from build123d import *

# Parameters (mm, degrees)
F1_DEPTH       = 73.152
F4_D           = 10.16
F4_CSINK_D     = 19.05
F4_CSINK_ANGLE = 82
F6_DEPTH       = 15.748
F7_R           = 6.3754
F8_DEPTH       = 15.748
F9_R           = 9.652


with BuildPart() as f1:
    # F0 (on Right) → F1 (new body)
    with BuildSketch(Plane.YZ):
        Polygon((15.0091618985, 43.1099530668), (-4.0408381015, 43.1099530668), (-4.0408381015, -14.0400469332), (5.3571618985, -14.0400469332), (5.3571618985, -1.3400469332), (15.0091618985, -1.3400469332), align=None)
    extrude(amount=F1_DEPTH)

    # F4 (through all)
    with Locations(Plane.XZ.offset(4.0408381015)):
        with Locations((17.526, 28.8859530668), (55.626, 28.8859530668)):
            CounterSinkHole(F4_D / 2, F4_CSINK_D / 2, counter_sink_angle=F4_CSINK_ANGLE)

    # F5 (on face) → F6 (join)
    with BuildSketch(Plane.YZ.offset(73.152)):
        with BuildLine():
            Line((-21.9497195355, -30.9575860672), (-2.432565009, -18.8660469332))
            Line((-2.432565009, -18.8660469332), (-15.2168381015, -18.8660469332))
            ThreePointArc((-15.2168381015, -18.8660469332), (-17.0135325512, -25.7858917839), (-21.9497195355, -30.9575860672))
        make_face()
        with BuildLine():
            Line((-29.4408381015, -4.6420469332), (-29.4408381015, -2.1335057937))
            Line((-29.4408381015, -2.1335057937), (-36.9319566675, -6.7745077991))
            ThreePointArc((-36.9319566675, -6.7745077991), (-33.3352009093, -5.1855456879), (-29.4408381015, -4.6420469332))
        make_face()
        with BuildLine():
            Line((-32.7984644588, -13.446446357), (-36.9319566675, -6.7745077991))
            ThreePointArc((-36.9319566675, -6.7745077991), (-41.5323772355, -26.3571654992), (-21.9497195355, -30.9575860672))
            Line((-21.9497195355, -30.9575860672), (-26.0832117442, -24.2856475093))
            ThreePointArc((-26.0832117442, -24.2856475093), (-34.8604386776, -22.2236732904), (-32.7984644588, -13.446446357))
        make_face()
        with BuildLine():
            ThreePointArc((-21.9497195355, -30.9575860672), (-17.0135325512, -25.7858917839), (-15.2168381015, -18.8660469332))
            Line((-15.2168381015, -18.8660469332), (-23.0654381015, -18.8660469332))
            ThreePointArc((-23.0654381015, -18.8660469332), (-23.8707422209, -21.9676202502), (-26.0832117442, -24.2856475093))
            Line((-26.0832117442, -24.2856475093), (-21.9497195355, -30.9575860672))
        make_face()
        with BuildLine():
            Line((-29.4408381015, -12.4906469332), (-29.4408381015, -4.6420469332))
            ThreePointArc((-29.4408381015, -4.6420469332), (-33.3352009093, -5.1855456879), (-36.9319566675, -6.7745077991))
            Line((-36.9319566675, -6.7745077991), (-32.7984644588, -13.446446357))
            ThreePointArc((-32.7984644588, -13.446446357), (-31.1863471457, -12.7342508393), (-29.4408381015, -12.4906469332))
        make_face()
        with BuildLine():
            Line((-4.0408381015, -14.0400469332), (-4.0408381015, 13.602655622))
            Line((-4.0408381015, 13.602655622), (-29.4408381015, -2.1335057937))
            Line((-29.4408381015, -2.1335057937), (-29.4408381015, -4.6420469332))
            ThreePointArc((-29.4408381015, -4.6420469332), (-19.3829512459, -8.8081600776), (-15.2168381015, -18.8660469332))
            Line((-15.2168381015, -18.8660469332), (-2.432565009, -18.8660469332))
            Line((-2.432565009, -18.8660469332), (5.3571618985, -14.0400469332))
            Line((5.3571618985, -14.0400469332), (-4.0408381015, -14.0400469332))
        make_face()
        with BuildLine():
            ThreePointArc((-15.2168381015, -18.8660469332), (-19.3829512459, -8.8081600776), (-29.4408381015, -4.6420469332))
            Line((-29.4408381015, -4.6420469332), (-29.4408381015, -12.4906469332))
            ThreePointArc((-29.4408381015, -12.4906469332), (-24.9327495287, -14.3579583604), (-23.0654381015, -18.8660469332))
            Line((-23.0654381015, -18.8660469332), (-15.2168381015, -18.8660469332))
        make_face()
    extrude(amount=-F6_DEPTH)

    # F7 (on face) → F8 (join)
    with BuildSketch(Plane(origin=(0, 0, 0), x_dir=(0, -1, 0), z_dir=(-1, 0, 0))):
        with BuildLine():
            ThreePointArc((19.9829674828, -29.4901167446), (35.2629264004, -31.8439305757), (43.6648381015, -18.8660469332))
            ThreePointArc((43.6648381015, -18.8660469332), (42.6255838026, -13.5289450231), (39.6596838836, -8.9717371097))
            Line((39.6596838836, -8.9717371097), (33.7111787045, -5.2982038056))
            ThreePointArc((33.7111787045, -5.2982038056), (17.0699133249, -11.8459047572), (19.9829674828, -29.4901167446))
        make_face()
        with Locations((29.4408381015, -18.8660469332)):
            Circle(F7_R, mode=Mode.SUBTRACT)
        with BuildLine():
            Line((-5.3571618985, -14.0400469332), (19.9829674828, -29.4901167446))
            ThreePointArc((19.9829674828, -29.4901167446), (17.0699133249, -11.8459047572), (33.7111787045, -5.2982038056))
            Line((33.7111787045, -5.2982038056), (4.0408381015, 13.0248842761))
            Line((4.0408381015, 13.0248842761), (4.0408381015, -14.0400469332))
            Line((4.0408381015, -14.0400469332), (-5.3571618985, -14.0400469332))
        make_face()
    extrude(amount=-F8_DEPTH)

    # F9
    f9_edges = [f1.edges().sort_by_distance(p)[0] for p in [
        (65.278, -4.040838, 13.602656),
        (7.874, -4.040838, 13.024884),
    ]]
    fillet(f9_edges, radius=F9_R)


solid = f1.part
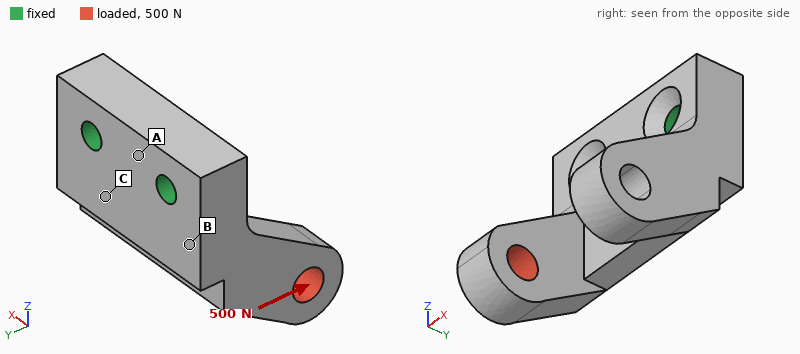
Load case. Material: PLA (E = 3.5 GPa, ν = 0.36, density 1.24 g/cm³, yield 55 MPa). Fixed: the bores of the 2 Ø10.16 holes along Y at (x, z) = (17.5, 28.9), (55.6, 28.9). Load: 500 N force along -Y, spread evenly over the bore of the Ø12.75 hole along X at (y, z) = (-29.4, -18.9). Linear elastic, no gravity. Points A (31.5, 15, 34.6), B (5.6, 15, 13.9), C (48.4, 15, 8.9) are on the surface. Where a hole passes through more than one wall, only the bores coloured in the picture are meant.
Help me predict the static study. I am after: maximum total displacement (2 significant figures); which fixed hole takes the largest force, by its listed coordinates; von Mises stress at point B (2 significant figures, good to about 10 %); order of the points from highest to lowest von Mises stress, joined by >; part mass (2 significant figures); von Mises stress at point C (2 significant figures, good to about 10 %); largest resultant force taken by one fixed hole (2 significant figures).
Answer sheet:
0.71 mm
(17.5, 28.9)
6.6 MPa
B > C > A
120 g
2.7 MPa
520 N
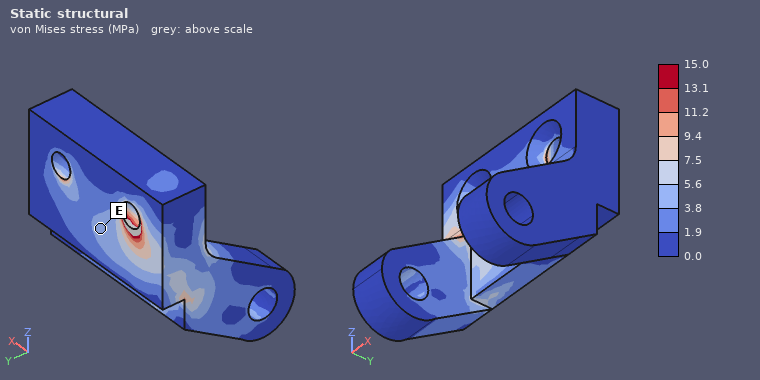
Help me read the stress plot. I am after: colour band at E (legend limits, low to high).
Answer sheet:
3.8 to 5.6 MPa
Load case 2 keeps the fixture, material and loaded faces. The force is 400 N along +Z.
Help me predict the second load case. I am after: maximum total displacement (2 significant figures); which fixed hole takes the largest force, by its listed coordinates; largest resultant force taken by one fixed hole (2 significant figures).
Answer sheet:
0.57 mm
(17.5, 28.9)
450 N
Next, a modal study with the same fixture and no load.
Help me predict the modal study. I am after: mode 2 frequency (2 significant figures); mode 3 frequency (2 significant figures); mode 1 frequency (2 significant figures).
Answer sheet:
1100 Hz
1400 Hz
970 Hz
